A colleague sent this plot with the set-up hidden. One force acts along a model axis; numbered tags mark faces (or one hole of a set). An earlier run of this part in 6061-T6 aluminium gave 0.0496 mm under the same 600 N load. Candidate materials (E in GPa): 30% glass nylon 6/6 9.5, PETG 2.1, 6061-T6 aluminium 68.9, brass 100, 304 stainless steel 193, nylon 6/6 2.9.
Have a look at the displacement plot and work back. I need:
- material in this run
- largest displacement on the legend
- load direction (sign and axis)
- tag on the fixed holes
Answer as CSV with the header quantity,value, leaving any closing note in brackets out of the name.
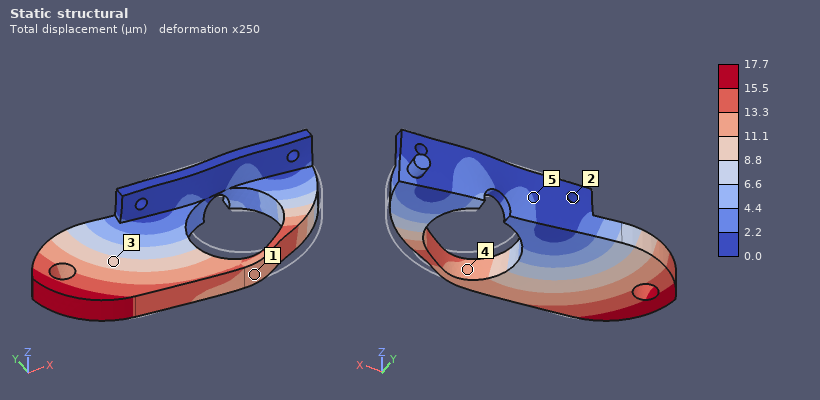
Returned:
quantity,value
material in this run,304 stainless steel
largest displacement on the legend,17.7 µm
load direction,-X
tag on the fixed holes,2
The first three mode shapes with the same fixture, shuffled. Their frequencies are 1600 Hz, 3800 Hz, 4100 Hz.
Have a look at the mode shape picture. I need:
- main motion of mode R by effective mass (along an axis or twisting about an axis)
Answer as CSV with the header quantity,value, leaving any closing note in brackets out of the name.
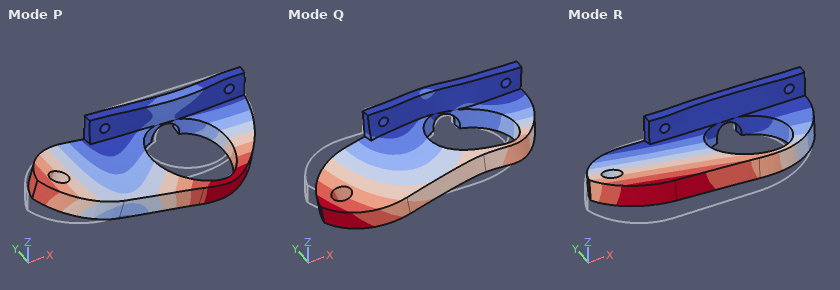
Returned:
quantity,value
main motion of mode R by effective mass,along Z
